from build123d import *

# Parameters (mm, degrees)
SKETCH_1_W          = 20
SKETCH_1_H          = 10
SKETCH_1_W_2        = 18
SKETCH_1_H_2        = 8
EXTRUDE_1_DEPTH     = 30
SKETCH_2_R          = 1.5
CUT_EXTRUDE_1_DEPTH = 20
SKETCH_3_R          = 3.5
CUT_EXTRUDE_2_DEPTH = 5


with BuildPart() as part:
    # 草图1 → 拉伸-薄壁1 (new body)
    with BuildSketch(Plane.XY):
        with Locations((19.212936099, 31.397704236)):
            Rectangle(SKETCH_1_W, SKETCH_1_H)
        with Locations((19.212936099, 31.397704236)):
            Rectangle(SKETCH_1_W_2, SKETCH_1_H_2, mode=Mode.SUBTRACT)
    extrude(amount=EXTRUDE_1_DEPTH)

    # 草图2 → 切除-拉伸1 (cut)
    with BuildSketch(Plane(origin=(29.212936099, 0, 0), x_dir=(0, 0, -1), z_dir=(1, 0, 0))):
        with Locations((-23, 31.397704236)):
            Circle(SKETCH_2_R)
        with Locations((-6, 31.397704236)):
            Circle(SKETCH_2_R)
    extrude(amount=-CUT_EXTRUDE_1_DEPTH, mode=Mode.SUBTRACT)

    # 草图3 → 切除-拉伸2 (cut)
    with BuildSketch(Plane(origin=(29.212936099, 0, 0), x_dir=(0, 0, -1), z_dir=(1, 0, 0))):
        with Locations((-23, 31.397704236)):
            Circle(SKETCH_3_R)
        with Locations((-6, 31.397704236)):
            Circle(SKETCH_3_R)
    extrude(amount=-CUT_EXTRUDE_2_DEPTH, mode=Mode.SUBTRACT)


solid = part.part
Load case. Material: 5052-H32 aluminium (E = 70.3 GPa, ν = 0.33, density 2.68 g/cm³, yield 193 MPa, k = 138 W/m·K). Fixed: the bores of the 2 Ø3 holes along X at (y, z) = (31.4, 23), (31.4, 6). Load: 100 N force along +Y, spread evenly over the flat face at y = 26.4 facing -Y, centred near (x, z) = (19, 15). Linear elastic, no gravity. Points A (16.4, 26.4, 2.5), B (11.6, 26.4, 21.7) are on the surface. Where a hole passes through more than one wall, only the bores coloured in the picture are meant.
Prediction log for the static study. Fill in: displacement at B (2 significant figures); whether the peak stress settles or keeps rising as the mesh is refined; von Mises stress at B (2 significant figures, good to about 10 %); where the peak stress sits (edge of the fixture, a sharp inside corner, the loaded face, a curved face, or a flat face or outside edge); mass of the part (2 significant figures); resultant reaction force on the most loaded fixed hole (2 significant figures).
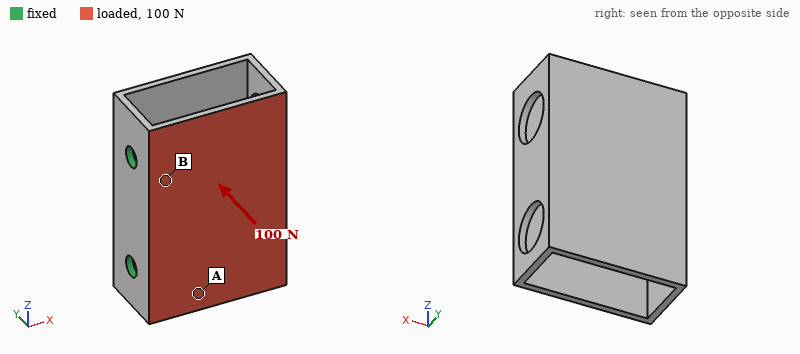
0.035 mm
keeps rising
39 MPa
edge of the fixture
4.3 g
52 N
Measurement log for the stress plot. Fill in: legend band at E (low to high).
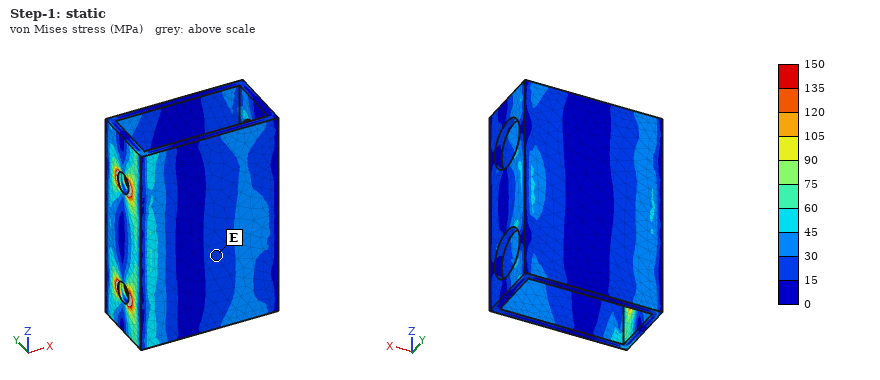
15 to 30 MPa
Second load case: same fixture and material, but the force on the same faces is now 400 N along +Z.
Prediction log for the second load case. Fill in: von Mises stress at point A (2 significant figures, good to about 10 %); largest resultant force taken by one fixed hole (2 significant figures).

27 MPa
300 N
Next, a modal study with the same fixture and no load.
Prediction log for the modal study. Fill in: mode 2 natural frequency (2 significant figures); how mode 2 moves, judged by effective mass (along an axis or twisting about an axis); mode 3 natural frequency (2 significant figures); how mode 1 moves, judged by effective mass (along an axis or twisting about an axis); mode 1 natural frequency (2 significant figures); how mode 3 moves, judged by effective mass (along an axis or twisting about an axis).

6200 Hz
twisting about X
7000 Hz
along Y
1900 Hz
along Z
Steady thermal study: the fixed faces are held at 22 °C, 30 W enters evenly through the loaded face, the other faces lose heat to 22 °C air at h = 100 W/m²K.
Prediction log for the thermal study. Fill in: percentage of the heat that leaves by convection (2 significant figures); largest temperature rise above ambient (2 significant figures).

25 %
56 K
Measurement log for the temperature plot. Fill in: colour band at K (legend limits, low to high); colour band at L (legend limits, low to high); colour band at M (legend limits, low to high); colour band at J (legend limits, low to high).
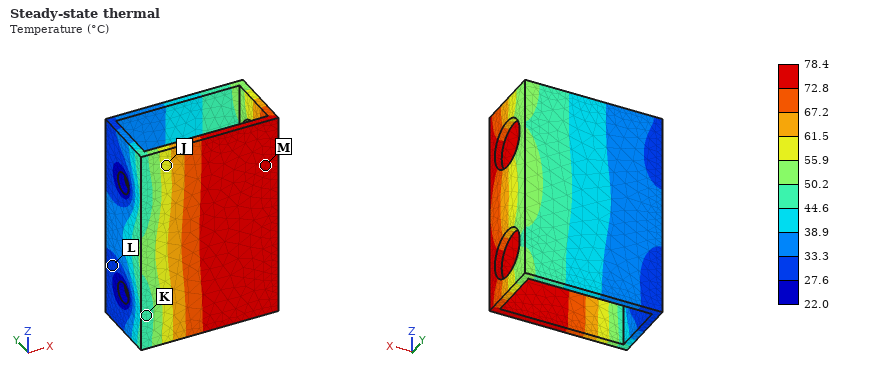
44.6 to 50.2 °C
27.6 to 33.3 °C
72.8 to 78.4 °C
55.9 to 61.5 °C
